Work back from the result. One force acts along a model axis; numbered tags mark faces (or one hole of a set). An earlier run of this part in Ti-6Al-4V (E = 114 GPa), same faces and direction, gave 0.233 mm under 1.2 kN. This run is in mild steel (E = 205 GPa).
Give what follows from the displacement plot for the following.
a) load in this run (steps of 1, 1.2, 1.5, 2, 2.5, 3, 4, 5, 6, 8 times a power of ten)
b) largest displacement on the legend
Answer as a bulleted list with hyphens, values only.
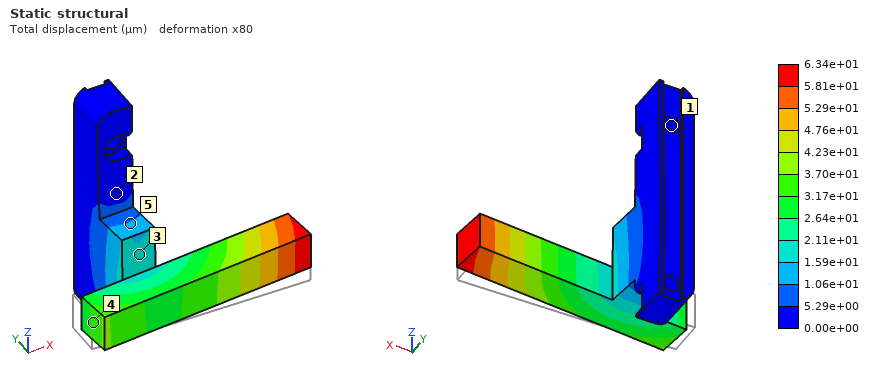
- 600 N
- 6.34e+01 µm
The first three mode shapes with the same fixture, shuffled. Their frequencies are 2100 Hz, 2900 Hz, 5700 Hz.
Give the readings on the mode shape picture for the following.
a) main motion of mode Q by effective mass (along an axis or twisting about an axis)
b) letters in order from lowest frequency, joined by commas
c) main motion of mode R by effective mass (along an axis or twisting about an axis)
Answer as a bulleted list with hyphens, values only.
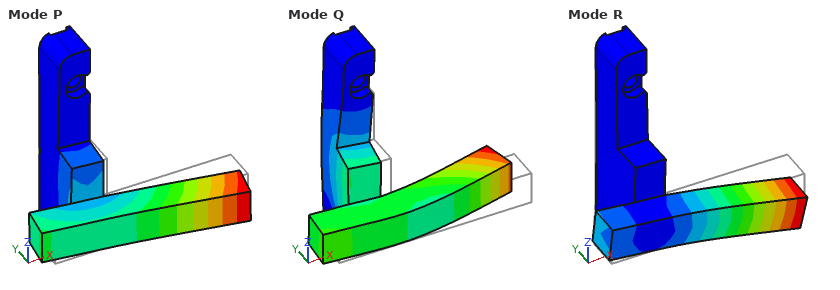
- along X
- P, R, Q
- along Z
